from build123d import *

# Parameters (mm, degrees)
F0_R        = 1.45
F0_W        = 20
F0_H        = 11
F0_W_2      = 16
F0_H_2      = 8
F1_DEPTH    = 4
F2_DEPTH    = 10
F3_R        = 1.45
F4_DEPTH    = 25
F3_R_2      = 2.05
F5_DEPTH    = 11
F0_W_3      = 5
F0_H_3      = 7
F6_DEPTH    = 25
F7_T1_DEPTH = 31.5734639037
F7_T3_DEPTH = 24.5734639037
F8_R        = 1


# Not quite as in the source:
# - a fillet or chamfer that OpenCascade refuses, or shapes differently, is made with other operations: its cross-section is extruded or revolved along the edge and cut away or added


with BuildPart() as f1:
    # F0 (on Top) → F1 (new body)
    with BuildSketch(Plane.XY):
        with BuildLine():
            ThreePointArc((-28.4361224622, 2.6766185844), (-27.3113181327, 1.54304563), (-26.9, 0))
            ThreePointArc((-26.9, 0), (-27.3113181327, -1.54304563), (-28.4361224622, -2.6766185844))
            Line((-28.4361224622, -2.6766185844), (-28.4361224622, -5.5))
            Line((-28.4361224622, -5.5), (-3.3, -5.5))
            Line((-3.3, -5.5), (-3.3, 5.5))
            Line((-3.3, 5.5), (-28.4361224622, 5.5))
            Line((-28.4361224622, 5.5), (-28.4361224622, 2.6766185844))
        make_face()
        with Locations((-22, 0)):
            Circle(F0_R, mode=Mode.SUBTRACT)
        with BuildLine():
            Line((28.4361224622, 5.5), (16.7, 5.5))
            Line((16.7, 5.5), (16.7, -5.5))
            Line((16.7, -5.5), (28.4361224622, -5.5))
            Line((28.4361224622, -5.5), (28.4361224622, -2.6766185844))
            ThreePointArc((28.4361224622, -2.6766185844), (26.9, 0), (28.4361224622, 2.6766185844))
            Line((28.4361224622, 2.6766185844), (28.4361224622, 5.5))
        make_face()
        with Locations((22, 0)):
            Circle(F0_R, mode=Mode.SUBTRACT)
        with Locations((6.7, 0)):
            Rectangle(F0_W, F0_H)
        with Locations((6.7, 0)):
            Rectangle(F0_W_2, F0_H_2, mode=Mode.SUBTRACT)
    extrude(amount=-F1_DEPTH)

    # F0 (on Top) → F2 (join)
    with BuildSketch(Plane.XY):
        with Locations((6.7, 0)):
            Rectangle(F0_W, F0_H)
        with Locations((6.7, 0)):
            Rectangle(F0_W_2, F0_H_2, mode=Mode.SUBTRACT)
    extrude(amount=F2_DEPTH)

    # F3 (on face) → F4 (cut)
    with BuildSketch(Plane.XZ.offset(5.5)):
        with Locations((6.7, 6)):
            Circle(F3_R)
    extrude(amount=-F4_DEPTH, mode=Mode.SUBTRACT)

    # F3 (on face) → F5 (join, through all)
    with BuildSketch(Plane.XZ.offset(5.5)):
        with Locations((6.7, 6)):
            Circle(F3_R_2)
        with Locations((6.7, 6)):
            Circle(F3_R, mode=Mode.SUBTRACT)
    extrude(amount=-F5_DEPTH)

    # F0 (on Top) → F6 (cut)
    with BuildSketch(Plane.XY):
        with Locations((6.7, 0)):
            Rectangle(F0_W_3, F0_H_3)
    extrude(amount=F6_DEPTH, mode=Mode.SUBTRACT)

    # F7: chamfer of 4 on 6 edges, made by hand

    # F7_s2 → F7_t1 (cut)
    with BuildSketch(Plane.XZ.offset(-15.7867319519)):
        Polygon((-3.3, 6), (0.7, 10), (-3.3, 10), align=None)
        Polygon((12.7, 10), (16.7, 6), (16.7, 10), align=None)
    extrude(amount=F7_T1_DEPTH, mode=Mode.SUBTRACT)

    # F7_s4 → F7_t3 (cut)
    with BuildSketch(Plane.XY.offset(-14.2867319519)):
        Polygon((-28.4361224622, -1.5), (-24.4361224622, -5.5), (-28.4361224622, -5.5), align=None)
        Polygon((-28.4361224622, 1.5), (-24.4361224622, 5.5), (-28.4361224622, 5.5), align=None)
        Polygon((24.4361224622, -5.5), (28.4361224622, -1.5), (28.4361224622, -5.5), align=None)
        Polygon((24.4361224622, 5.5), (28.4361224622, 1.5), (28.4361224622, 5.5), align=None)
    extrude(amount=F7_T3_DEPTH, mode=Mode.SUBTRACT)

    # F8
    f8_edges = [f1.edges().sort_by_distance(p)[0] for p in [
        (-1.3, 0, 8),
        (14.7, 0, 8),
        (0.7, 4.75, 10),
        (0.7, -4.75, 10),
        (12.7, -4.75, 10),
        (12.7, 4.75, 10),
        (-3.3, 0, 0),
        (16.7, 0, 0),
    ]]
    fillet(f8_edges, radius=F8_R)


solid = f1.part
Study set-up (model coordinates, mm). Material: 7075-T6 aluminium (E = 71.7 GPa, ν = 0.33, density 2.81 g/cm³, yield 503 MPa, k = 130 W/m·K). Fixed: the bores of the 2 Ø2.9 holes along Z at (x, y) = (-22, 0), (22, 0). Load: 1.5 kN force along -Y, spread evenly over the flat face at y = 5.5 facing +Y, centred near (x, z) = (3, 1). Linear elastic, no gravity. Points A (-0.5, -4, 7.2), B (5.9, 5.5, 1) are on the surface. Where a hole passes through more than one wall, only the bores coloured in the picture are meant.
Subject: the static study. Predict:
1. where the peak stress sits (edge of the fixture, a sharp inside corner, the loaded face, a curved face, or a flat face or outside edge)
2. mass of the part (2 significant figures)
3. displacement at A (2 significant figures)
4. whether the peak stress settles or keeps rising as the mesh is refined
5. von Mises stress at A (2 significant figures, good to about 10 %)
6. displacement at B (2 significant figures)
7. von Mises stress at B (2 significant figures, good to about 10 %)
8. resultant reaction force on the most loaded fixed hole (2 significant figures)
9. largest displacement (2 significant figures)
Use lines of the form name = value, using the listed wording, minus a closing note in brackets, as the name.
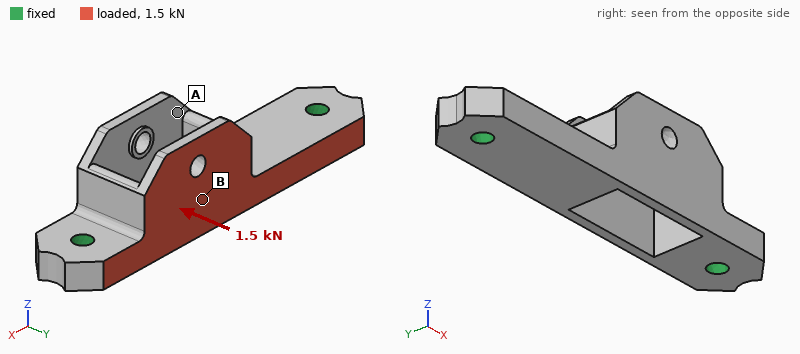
where the peak stress sits = a sharp inside corner
mass of the part = 7.1 g
displacement at A = 0.12 mm
whether the peak stress settles or keeps rising as the mesh is refined = keeps rising
von Mises stress at A = 47 MPa
displacement at B = 0.12 mm
von Mises stress at B = 190 MPa
resultant reaction force on the most loaded fixed hole = 770 N
largest displacement = 0.23 mm
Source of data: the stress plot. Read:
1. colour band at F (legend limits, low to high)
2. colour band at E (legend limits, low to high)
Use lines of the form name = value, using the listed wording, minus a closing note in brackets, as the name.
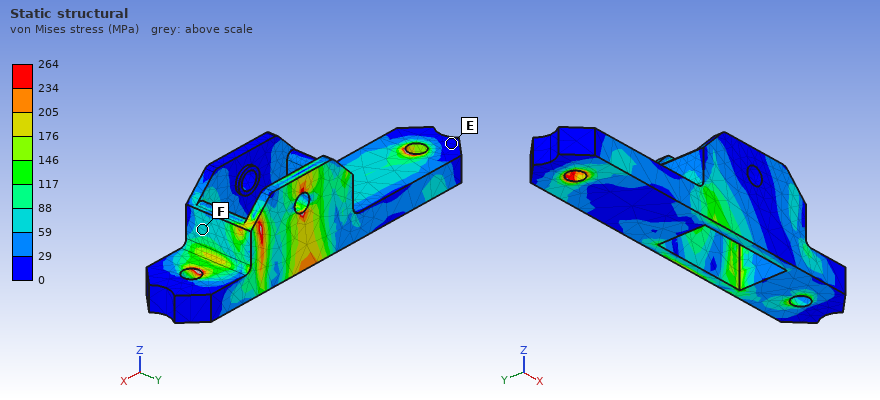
colour band at F = 59 to 88 MPa
colour band at E = 0 to 29 MPa
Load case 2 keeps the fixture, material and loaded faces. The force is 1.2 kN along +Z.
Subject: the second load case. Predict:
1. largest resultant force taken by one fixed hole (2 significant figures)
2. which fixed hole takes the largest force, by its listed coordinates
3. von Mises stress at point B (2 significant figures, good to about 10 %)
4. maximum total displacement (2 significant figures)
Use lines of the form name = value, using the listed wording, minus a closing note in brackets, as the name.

largest resultant force taken by one fixed hole = 730 N
which fixed hole takes the largest force, by its listed coordinates = (22, 0)
von Mises stress at point B = 40 MPa
maximum total displacement = 0.15 mm
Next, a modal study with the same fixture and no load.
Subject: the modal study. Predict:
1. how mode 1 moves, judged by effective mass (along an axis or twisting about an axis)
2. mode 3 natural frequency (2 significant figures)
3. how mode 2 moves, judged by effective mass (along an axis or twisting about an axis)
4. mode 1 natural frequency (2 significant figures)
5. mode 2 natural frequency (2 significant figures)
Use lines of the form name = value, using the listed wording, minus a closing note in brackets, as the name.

how mode 1 moves, judged by effective mass = along Y
mode 3 natural frequency = 14 kHz
how mode 2 moves, judged by effective mass = along Z
mode 1 natural frequency = 9100 Hz
mode 2 natural frequency = 10 kHz
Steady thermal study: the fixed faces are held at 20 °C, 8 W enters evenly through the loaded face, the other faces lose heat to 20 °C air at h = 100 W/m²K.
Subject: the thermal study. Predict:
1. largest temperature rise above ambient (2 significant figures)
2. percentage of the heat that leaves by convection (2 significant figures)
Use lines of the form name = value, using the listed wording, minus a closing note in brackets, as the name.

largest temperature rise above ambient = 14 K
percentage of the heat that leaves by convection = 14 %
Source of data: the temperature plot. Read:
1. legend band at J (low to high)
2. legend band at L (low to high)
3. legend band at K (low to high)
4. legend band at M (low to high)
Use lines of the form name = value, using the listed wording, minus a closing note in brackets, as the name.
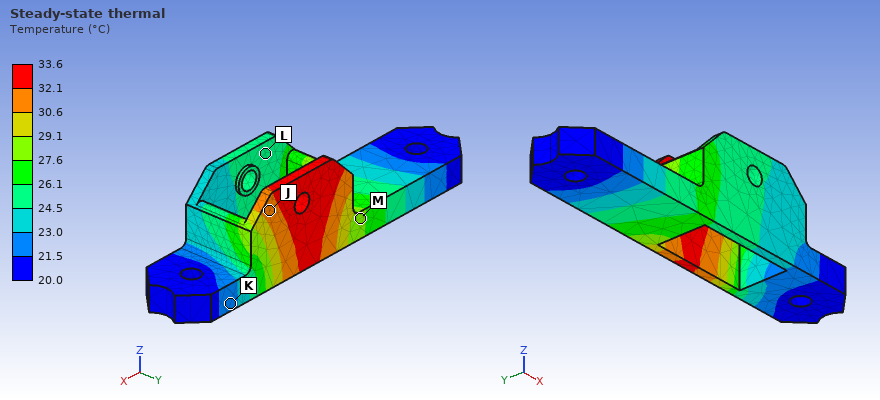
legend band at J = 30.6 to 32.1 °C
legend band at L = 24.5 to 26.1 °C
legend band at K = 21.5 to 23.0 °C
legend band at M = 27.6 to 29.1 °C
